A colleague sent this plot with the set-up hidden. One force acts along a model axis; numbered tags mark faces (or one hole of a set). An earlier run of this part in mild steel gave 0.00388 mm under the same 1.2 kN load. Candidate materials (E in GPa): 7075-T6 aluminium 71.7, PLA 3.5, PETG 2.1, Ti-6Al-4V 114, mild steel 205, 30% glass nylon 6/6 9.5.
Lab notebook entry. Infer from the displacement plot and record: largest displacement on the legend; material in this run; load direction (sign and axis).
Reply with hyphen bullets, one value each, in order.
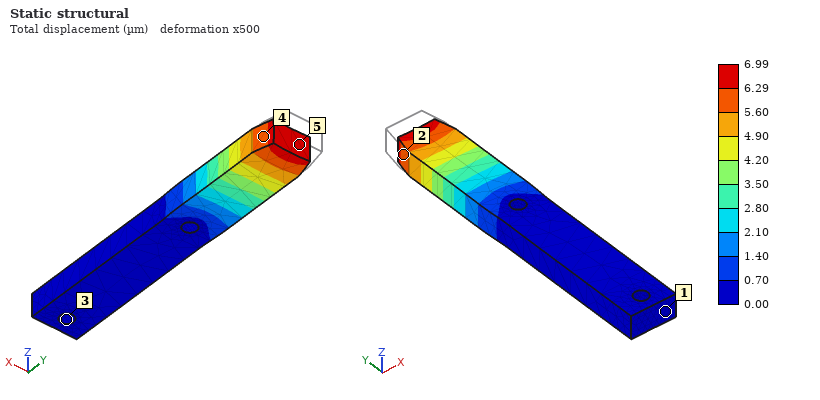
- 6.99 µm
- Ti-6Al-4V
- -Y
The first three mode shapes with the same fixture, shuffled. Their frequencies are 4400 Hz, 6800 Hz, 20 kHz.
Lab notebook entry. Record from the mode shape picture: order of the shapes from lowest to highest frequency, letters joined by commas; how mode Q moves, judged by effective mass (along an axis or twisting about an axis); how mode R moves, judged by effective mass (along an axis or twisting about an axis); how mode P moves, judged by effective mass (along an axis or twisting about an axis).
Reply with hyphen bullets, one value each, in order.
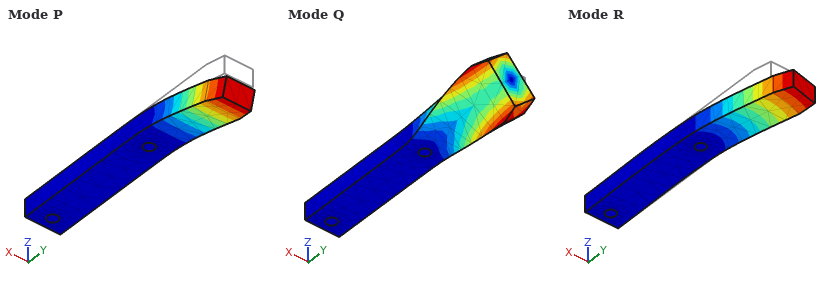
- P, R, Q
- twisting about Y
- along X
- along Z
